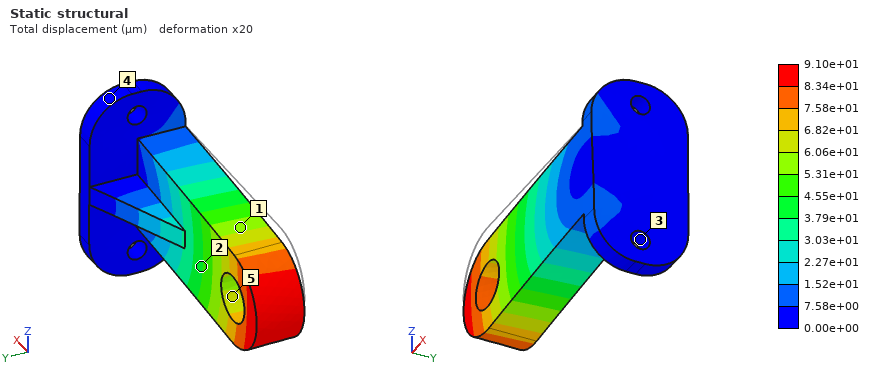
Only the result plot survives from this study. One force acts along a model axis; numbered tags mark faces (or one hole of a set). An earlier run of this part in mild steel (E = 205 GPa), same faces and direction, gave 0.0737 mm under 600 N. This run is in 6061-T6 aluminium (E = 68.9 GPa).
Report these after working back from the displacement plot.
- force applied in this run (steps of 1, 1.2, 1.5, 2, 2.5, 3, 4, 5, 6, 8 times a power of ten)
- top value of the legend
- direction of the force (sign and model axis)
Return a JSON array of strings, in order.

["250 N", "9.10e+01 µm", "-Z"]
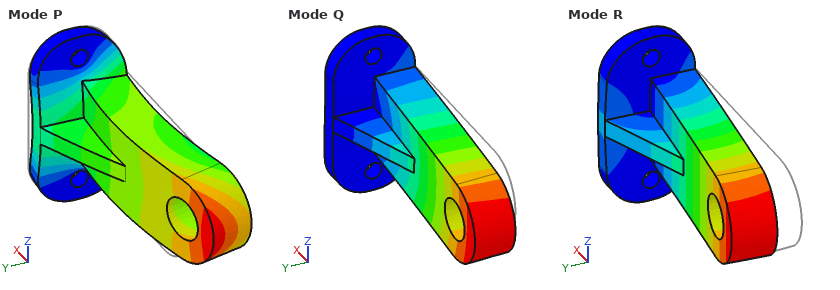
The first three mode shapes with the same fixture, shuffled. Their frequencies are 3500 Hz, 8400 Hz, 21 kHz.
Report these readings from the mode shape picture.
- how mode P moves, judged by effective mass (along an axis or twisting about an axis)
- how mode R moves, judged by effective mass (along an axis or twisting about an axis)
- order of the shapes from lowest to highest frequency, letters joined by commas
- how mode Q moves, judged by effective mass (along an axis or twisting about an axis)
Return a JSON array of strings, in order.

["along X", "along Y", "R, Q, P", "along Z"]
